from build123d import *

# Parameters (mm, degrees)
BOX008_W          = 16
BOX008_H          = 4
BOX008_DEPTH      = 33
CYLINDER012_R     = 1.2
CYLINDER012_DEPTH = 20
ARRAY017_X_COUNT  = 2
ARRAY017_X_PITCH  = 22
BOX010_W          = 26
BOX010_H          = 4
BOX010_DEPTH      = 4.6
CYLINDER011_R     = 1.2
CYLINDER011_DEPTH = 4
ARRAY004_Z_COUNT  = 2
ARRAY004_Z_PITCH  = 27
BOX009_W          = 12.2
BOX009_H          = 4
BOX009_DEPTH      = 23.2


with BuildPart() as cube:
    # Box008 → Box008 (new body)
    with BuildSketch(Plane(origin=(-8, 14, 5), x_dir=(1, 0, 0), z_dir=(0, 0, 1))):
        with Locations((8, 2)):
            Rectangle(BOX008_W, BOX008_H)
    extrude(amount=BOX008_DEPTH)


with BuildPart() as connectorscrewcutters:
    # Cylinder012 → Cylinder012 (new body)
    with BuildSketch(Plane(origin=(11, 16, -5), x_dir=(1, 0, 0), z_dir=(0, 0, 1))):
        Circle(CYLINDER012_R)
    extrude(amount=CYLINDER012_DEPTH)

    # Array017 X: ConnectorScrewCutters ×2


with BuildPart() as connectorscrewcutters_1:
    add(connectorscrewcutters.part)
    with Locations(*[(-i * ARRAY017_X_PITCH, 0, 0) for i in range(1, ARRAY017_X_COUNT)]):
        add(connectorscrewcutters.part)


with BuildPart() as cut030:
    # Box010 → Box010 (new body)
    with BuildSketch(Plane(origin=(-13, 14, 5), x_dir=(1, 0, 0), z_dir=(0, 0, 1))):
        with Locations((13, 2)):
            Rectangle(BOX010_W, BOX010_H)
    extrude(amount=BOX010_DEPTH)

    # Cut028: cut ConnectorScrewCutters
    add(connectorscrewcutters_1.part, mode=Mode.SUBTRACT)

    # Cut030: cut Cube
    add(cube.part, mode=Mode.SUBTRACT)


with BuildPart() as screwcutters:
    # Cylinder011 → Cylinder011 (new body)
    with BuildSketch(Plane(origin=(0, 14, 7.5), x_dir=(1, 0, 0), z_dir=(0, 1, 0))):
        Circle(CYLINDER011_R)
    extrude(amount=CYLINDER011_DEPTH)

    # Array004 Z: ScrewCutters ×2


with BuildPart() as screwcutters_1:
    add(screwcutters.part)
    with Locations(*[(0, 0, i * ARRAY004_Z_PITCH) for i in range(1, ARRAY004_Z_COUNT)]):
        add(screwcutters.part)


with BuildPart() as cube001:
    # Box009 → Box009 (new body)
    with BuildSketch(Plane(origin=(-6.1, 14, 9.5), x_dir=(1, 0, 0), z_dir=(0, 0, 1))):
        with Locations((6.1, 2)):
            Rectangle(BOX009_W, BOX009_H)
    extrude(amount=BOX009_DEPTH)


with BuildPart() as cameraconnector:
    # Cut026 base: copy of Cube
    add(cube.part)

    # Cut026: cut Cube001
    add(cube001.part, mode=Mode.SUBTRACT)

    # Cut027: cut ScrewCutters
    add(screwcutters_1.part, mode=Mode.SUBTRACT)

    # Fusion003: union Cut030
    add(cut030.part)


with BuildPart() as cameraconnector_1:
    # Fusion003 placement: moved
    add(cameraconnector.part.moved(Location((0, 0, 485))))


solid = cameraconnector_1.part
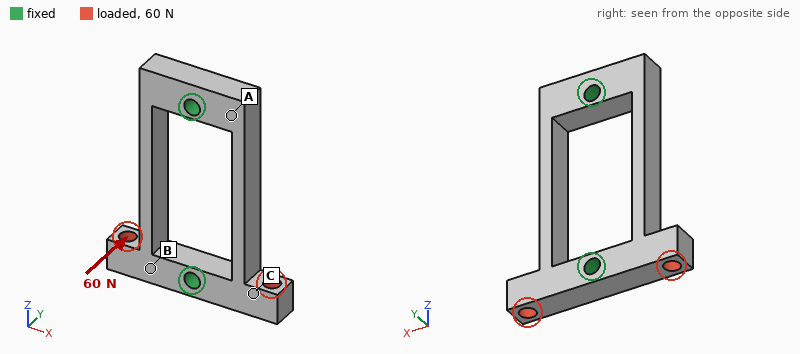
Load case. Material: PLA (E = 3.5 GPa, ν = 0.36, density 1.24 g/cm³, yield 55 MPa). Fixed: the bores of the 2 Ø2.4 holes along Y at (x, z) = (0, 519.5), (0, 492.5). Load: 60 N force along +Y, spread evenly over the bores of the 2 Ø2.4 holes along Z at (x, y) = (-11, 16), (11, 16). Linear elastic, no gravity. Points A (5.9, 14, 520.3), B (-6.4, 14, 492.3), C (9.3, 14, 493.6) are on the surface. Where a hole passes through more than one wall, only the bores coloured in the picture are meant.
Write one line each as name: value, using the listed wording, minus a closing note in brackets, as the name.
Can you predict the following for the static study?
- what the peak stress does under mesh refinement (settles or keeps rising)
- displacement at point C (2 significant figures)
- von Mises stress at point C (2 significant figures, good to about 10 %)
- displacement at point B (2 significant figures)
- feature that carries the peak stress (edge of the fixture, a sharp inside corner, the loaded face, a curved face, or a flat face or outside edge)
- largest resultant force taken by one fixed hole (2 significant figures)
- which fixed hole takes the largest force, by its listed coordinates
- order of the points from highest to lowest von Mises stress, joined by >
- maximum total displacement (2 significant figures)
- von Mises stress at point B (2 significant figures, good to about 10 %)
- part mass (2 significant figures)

what the peak stress does under mesh refinement: keeps rising
displacement at point C: 0.11 mm
von Mises stress at point C: 7.7 MPa
displacement at point B: 0.062 mm
feature that carries the peak stress: edge of the fixture
largest resultant force taken by one fixed hole: 59 N
which fixed hole takes the largest force, by its listed coordinates: (0, 492.5)
order of the points from highest to lowest von Mises stress, joined by >: B > C > A
maximum total displacement: 0.19 mm
von Mises stress at point B: 11 MPa
part mass: 1.3 g
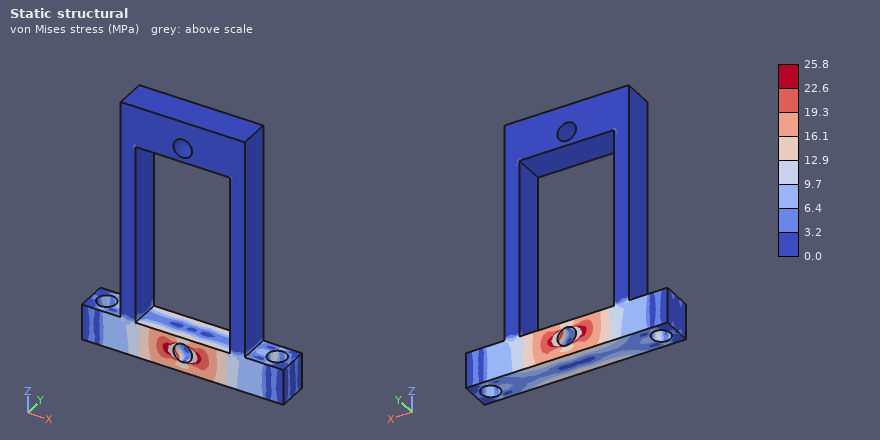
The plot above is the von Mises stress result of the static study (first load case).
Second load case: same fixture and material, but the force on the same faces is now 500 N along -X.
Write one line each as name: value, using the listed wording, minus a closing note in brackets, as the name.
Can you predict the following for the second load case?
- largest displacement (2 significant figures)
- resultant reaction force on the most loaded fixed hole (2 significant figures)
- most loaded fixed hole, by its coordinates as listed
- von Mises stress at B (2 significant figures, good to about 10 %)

largest displacement: 73 µm
resultant reaction force on the most loaded fixed hole: 500 N
most loaded fixed hole, by its coordinates as listed: (0, 492.5)
von Mises stress at B: 15 MPa
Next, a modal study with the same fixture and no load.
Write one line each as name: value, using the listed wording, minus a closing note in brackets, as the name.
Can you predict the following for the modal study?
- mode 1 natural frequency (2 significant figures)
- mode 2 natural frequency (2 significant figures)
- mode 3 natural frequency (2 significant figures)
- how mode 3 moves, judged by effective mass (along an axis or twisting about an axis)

mode 1 natural frequency: 4900 Hz
mode 2 natural frequency: 4900 Hz
mode 3 natural frequency: 5700 Hz
how mode 3 moves, judged by effective mass: twisting about Z
